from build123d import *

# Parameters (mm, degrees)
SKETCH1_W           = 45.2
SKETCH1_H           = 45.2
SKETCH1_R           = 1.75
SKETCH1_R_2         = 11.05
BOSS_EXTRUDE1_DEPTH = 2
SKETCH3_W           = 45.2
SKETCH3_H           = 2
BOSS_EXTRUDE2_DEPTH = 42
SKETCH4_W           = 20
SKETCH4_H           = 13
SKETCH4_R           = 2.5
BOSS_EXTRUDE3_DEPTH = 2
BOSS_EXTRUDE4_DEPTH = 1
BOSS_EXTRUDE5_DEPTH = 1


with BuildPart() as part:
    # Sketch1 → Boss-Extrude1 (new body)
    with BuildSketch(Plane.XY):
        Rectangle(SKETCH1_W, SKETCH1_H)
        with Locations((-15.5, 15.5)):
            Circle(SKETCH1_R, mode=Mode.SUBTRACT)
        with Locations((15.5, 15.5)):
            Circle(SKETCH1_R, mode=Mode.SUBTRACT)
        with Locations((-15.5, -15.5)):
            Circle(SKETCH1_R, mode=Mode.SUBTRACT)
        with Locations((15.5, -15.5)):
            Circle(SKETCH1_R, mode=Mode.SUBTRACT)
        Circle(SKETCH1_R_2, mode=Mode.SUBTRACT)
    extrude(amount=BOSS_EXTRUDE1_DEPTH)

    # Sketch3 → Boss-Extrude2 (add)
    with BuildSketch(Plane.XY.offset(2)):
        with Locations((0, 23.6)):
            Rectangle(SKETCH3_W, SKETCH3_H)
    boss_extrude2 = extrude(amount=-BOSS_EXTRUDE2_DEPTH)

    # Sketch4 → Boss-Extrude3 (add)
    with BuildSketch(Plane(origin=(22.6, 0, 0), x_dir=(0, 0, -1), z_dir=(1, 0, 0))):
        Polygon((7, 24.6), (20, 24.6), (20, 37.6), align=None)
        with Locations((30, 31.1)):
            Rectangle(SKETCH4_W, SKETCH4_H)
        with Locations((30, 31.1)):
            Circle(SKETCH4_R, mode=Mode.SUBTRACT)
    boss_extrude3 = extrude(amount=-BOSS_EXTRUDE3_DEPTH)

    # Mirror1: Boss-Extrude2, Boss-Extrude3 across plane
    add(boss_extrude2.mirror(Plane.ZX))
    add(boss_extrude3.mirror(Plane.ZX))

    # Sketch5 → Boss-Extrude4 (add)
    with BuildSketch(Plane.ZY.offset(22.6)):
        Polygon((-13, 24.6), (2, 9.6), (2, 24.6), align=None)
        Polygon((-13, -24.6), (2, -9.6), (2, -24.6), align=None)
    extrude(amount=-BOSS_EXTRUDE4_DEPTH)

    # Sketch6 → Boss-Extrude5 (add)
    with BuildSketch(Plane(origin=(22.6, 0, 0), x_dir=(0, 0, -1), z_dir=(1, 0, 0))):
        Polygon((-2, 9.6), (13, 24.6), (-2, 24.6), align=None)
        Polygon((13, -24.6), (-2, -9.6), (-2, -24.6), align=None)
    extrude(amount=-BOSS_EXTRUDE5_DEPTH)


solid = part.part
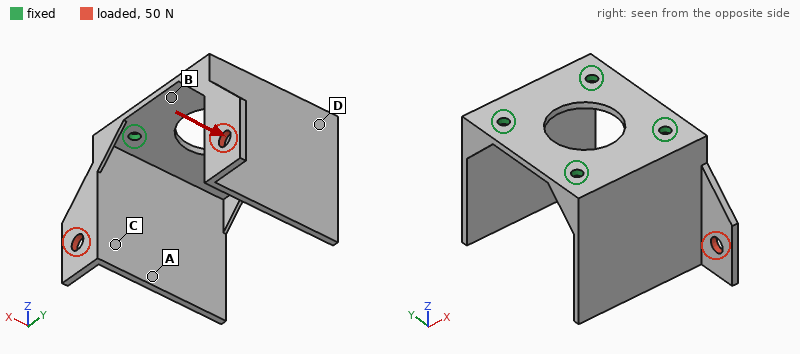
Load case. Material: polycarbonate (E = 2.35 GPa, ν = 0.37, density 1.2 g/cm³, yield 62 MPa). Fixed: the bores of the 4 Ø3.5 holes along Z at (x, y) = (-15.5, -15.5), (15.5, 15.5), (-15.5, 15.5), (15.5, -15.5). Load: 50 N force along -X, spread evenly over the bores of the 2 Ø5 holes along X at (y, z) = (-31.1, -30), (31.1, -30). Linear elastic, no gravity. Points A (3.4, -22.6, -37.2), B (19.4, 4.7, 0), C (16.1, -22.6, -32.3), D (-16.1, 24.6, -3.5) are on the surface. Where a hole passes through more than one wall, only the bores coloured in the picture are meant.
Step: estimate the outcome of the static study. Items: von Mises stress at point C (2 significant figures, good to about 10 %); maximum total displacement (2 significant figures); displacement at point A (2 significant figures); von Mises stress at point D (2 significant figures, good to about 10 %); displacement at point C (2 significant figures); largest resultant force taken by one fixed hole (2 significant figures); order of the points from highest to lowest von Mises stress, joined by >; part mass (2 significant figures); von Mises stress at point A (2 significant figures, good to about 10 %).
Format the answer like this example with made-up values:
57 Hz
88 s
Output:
6.6 MPa
1.0 mm
0.44 mm
2.4 MPa
0.17 mm
28 N
C > A > D > B
15 g
3.6 MPa
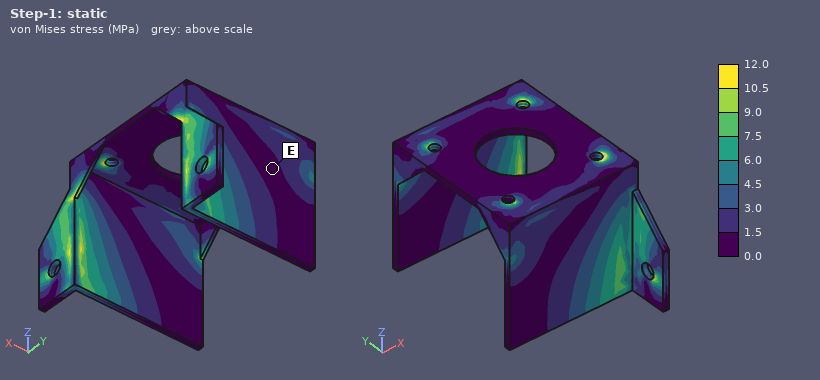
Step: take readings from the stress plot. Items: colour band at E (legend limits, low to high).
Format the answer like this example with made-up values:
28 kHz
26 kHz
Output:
0.0 to 1.5 MPa
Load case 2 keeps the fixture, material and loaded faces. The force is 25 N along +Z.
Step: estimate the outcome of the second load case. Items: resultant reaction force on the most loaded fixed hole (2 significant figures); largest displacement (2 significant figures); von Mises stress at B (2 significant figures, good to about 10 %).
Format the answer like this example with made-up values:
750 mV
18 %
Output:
15 N
1.1 mm
1.2 MPa
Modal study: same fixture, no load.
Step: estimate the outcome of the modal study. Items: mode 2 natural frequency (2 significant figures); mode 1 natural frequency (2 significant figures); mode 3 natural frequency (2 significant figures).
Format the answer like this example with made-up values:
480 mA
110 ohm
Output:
260 Hz
260 Hz
530 Hz
